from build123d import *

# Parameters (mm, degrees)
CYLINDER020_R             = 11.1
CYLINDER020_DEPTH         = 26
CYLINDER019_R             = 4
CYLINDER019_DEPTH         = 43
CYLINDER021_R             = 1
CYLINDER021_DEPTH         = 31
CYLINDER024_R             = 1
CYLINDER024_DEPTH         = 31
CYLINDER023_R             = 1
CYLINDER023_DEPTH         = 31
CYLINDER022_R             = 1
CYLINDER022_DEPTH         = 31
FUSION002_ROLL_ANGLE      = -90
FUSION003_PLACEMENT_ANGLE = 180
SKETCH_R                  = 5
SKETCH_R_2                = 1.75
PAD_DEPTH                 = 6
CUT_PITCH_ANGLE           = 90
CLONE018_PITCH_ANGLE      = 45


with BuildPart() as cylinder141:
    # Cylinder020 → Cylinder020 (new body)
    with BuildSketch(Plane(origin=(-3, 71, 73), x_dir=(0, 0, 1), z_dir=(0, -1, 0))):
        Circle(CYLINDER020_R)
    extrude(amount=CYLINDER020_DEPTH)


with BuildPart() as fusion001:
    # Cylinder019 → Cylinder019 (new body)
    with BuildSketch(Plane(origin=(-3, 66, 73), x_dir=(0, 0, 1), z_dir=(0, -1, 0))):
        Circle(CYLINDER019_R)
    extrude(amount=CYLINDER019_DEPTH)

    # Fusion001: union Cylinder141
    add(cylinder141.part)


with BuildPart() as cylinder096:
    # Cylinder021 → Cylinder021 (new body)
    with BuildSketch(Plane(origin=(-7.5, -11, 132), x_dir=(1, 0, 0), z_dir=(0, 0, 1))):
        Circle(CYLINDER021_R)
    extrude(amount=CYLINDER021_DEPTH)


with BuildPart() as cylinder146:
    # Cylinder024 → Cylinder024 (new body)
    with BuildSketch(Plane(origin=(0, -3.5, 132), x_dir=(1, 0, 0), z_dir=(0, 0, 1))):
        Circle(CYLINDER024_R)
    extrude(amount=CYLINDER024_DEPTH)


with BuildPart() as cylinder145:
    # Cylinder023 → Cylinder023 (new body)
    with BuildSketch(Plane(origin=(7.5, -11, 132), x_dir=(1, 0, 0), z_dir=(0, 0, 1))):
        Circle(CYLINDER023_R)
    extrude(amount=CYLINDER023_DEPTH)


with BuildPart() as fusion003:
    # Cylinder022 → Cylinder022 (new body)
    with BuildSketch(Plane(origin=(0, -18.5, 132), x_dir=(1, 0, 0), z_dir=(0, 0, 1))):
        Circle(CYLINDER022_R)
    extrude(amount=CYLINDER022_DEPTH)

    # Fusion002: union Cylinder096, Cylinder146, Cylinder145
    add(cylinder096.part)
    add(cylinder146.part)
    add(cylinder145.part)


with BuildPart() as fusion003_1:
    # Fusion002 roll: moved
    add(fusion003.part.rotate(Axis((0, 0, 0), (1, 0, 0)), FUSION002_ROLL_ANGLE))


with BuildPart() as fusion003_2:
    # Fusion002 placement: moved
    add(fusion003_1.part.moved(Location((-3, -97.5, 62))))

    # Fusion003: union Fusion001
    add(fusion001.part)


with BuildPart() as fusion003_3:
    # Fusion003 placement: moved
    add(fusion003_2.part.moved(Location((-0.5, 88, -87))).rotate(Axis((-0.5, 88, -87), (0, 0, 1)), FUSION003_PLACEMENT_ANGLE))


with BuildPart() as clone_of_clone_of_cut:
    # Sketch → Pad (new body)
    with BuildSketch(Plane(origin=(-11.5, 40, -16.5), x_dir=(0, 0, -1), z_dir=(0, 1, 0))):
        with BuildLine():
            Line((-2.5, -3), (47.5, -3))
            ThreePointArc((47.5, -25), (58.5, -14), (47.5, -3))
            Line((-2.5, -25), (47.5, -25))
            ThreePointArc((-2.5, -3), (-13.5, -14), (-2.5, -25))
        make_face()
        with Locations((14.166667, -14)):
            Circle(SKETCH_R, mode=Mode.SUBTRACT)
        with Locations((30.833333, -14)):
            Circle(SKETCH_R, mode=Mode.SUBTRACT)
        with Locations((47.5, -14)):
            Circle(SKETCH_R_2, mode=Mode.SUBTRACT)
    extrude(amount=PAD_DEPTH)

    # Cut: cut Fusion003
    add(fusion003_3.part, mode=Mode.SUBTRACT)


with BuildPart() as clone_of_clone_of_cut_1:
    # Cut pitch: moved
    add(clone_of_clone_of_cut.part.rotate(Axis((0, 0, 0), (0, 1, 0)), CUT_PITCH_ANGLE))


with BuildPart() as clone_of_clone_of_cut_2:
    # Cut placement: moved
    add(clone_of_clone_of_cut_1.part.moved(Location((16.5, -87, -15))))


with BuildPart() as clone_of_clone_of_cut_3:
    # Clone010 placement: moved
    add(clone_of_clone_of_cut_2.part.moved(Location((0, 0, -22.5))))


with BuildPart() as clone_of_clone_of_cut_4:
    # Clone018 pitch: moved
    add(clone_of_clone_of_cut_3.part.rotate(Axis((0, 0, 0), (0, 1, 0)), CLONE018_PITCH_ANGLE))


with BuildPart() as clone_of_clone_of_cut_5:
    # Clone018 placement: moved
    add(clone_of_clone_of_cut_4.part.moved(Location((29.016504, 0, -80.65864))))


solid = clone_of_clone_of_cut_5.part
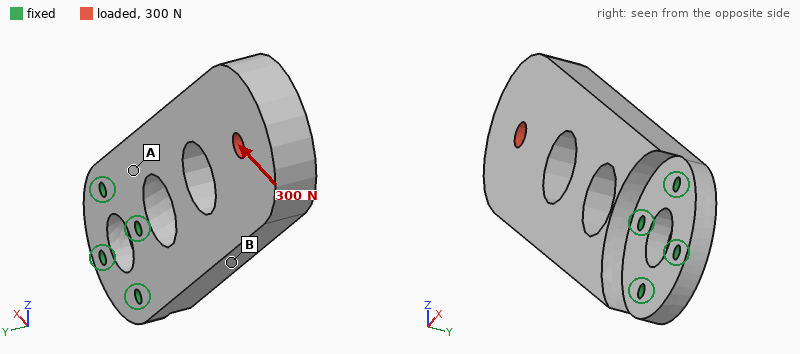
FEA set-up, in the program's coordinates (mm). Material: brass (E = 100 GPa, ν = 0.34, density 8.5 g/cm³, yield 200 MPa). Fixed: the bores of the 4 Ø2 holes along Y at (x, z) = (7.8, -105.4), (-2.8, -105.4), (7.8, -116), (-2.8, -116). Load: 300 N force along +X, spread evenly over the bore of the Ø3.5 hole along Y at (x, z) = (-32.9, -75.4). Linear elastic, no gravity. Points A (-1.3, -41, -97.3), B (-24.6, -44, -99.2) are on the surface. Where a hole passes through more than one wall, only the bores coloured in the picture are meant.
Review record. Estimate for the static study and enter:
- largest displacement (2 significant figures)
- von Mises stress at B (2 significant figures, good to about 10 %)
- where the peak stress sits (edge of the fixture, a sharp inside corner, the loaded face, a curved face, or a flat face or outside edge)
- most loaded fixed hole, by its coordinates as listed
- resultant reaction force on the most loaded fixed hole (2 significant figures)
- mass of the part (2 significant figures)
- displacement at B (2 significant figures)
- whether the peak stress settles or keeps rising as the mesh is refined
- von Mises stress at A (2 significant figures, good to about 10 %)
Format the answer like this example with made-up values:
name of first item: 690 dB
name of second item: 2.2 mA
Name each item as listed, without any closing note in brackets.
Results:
largest displacement: 41 µm
von Mises stress at B: 10 MPa
where the peak stress sits: edge of the fixture
most loaded fixed hole, by its coordinates as listed: (7.8, -105.4)
resultant reaction force on the most loaded fixed hole: 540 N
mass of the part: 56 g
displacement at B: 13 µm
whether the peak stress settles or keeps rising as the mesh is refined: keeps rising
von Mises stress at A: 22 MPa
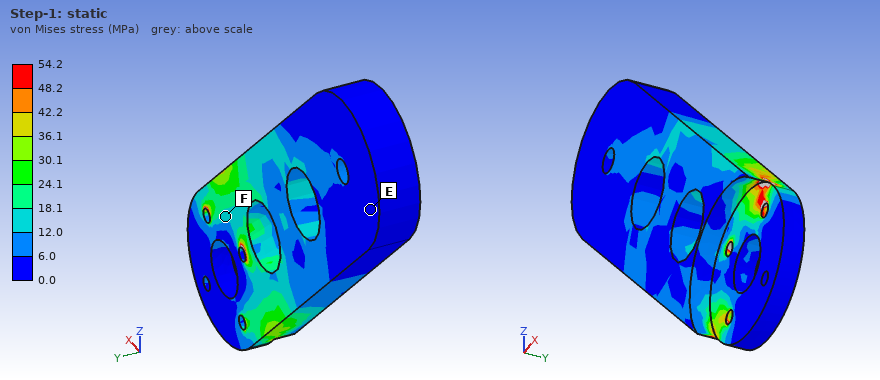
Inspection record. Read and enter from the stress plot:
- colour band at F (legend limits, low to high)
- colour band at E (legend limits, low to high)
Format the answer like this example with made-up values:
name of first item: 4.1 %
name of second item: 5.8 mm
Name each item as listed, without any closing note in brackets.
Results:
colour band at F: 12.0 to 18.1 MPa
colour band at E: 0.0 to 6.0 MPa
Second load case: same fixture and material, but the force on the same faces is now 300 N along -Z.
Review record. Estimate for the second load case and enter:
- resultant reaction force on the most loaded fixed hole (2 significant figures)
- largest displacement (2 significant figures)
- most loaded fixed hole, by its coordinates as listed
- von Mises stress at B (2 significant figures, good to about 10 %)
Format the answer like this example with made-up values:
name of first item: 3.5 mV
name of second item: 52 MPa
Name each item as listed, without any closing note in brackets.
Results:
resultant reaction force on the most loaded fixed hole: 540 N
largest displacement: 40 µm
most loaded fixed hole, by its coordinates as listed: (-2.8, -116)
von Mises stress at B: 17 MPa
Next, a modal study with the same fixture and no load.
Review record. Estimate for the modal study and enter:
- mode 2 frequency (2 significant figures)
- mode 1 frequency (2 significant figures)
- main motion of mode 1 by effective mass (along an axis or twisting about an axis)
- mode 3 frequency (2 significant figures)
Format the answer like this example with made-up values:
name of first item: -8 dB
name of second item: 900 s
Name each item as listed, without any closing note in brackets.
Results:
mode 2 frequency: 2600 Hz
mode 1 frequency: 730 Hz
main motion of mode 1 by effective mass: along Y
mode 3 frequency: 3300 Hz
